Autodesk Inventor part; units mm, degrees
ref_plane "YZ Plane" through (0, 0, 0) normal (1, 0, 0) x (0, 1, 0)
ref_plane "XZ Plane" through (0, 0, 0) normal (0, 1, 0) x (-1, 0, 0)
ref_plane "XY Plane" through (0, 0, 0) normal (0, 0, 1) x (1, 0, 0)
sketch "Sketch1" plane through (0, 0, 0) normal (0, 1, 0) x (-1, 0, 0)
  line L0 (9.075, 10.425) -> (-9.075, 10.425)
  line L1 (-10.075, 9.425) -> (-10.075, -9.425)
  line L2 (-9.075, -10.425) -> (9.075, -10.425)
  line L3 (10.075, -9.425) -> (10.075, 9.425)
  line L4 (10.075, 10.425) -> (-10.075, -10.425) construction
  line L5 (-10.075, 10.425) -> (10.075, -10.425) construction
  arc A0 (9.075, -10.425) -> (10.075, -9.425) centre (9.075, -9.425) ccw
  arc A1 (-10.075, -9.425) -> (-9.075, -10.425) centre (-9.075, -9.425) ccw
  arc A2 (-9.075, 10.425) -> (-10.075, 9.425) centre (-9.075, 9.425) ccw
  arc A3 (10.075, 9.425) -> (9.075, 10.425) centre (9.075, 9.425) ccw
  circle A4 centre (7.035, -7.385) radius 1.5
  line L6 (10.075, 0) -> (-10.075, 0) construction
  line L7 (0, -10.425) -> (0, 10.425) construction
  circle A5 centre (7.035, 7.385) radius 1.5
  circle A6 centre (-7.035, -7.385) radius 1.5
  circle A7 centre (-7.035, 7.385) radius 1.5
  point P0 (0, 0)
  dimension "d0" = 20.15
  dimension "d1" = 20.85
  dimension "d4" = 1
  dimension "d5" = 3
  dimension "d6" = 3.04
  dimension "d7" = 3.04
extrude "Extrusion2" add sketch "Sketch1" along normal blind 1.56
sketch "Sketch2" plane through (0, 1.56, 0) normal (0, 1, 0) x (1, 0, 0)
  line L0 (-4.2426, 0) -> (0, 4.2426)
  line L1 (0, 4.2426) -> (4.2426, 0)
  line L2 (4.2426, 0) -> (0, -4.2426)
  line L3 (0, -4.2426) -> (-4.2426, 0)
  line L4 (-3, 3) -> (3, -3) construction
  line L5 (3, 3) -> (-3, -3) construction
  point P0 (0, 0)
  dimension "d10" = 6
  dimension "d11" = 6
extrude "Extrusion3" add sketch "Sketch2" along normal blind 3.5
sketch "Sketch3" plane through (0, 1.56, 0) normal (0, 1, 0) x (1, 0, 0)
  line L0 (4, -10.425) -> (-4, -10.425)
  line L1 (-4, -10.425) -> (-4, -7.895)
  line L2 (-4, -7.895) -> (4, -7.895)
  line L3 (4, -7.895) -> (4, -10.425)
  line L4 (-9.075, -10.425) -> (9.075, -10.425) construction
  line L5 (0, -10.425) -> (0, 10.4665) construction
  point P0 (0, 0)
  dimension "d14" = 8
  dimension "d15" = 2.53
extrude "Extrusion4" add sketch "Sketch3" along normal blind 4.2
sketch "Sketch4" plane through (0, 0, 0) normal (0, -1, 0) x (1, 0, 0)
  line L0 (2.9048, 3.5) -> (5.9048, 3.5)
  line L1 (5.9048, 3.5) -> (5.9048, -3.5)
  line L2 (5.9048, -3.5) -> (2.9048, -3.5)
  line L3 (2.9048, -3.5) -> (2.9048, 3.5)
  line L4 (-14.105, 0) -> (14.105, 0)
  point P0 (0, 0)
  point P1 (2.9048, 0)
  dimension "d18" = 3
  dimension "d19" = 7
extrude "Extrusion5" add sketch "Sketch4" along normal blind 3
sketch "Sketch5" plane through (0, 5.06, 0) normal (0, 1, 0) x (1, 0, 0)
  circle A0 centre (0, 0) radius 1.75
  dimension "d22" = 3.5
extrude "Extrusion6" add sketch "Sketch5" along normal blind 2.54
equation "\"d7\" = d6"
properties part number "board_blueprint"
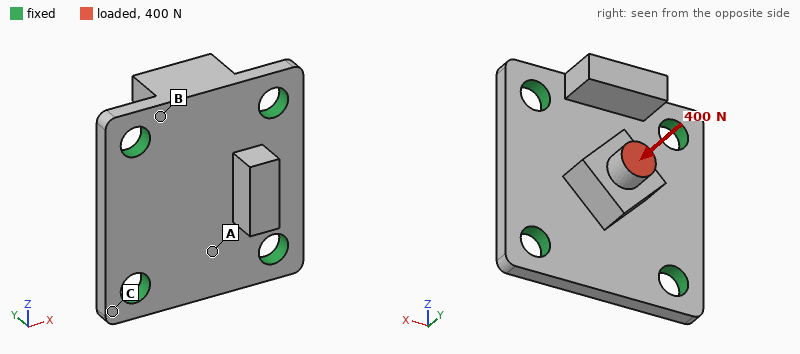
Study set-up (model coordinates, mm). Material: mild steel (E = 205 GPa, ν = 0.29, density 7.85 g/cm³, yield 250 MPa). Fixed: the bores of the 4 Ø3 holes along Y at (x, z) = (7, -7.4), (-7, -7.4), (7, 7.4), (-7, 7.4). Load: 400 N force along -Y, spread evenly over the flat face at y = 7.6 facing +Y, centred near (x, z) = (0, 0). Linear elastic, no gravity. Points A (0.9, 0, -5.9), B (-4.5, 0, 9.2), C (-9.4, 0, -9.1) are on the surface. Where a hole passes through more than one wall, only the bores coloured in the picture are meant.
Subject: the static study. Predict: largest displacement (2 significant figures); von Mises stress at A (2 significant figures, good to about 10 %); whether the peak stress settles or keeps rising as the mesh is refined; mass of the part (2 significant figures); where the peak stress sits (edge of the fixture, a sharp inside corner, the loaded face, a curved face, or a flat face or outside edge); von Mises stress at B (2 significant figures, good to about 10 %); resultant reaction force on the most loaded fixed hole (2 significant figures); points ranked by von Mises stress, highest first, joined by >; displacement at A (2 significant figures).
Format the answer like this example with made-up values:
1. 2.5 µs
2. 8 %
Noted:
1. 6.0 µm
2. 36 MPa
3. keeps rising
4. 7.1 g
5. edge of the fixture
6. 27 MPa
7. 100 N
8. A > B > C
9. 3.0 µm
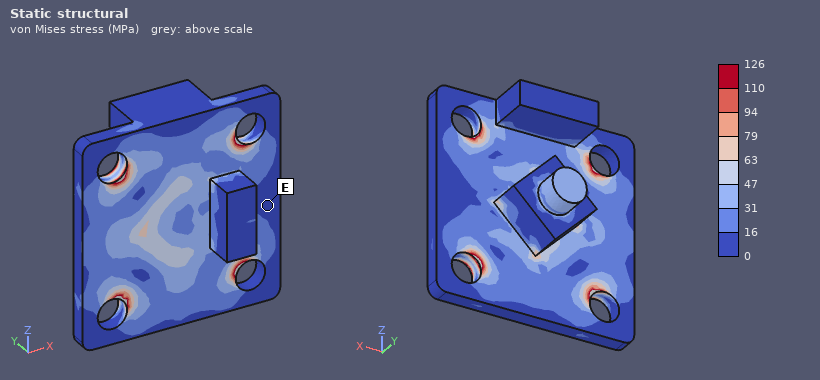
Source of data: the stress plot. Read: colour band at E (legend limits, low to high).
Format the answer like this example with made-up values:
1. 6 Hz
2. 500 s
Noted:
1. 0 to 16 MPa
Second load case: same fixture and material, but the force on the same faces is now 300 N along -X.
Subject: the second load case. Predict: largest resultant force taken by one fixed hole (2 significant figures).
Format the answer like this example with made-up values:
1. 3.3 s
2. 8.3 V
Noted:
1. 130 N
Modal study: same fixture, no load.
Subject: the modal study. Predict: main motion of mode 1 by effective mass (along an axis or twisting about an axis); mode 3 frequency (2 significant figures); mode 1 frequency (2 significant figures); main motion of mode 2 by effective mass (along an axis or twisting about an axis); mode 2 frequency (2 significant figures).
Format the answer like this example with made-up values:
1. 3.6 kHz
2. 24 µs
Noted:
1. along Y
2. 39 kHz
3. 27 kHz
4. along Y
5. 34 kHz
